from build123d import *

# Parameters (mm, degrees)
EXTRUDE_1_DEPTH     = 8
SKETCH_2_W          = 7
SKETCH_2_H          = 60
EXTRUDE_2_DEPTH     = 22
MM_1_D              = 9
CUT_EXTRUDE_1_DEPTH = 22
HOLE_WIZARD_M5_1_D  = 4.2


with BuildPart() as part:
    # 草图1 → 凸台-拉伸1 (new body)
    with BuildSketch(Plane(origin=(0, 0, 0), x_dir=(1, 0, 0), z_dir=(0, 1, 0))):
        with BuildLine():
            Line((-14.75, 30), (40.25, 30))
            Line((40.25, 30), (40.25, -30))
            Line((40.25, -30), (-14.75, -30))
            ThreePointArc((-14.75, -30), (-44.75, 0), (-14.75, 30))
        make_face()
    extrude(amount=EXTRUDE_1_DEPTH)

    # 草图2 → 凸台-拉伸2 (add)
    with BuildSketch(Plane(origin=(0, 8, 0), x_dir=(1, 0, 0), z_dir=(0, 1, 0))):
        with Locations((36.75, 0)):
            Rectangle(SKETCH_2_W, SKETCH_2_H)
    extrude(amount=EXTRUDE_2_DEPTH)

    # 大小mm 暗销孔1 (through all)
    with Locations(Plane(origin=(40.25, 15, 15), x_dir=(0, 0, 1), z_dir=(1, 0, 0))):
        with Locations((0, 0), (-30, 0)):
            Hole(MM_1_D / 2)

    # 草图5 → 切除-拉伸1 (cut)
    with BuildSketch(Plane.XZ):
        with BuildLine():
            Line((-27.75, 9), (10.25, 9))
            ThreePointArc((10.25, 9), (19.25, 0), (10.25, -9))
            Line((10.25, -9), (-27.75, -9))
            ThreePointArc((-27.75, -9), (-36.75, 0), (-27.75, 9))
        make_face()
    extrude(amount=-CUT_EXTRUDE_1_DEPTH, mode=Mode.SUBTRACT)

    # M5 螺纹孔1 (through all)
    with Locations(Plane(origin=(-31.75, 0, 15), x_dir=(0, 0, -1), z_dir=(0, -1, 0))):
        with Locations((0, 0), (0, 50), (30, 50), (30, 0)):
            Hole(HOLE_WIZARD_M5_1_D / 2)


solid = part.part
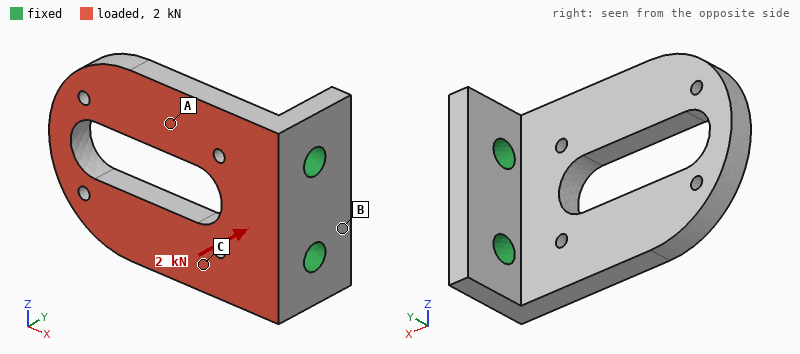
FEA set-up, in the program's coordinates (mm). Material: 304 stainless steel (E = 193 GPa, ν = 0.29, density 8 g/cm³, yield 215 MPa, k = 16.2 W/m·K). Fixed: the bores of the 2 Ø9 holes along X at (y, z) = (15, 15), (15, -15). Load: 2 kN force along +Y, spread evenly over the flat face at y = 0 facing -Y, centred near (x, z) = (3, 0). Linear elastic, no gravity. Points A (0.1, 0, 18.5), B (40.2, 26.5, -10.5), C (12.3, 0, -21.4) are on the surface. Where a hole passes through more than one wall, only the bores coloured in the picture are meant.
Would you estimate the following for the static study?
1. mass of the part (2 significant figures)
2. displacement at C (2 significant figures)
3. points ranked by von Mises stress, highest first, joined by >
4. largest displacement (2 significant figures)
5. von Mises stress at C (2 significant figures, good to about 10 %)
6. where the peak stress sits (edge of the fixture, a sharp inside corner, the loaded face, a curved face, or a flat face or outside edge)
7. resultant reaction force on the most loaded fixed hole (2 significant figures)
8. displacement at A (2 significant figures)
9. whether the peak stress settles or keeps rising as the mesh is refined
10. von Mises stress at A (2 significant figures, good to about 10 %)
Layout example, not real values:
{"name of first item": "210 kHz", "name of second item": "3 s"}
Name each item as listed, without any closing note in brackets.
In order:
{"mass of the part": "300 g", "displacement at C": "0.073 mm", "points ranked by von Mises stress, highest first, joined by >": "C > A > B", "largest displacement": "0.37 mm", "von Mises stress at C": "68 MPa", "where the peak stress sits": "edge of the fixture", "resultant reaction force on the most loaded fixed hole": "1.0 kN", "displacement at A": "0.13 mm", "whether the peak stress settles or keeps rising as the mesh is refined": "keeps rising", "von Mises stress at A": "41 MPa"}
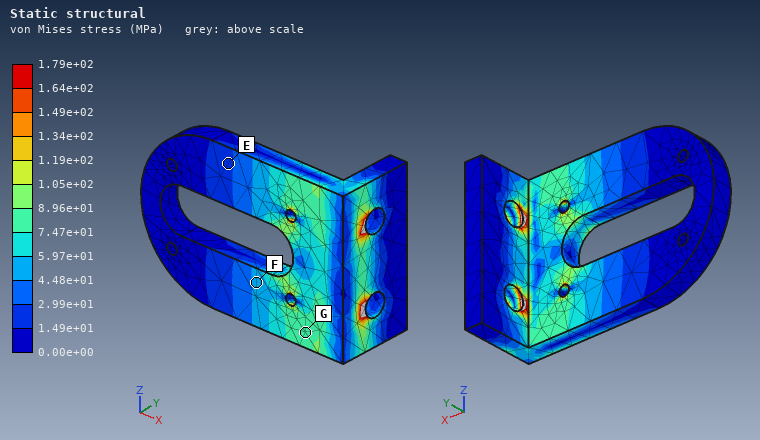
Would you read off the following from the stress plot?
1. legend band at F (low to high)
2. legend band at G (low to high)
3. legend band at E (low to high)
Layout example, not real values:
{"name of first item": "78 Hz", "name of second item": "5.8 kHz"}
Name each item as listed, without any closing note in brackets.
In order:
{"legend band at F": "4.48e+01 to 5.97e+01 MPa", "legend band at G": "7.47e+01 to 8.96e+01 MPa", "legend band at E": "1.49e+01 to 2.99e+01 MPa"}
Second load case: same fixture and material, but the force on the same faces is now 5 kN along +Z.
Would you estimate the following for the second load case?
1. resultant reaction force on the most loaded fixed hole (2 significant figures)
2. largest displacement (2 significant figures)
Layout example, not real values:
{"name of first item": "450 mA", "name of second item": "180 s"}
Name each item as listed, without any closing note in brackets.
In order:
{"resultant reaction force on the most loaded fixed hole": "5.4 kN", "largest displacement": "76 µm"}
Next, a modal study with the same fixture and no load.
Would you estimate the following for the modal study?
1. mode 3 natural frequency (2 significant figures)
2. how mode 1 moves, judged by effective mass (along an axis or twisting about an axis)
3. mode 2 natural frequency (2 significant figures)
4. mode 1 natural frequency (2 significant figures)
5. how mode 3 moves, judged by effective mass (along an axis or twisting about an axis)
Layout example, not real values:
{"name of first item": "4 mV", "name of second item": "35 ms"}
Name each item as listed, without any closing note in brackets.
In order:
{"mode 3 natural frequency": "3300 Hz", "how mode 1 moves, judged by effective mass": "along Y", "mode 2 natural frequency": "2600 Hz", "mode 1 natural frequency": "970 Hz", "how mode 3 moves, judged by effective mass": "along Z"}
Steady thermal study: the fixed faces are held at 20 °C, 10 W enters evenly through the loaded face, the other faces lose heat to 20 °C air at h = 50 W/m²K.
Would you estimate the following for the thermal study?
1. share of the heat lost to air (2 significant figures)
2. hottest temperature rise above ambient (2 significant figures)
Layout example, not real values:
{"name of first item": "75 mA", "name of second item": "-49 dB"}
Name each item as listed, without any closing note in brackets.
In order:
{"share of the heat lost to air": "55 %", "hottest temperature rise above ambient": "21 K"}
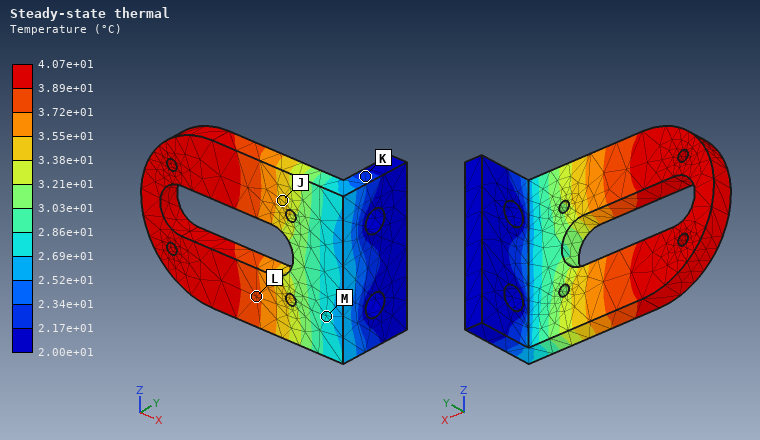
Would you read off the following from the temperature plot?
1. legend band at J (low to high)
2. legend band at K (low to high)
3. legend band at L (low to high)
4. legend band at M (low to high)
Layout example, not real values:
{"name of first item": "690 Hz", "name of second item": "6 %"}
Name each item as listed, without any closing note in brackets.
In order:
{"legend band at J": "3.38e+01 to 3.55e+01 °C", "legend band at K": "2.17e+01 to 2.34e+01 °C", "legend band at L": "3.72e+01 to 3.89e+01 °C", "legend band at M": "2.69e+01 to 2.86e+01 °C"}
